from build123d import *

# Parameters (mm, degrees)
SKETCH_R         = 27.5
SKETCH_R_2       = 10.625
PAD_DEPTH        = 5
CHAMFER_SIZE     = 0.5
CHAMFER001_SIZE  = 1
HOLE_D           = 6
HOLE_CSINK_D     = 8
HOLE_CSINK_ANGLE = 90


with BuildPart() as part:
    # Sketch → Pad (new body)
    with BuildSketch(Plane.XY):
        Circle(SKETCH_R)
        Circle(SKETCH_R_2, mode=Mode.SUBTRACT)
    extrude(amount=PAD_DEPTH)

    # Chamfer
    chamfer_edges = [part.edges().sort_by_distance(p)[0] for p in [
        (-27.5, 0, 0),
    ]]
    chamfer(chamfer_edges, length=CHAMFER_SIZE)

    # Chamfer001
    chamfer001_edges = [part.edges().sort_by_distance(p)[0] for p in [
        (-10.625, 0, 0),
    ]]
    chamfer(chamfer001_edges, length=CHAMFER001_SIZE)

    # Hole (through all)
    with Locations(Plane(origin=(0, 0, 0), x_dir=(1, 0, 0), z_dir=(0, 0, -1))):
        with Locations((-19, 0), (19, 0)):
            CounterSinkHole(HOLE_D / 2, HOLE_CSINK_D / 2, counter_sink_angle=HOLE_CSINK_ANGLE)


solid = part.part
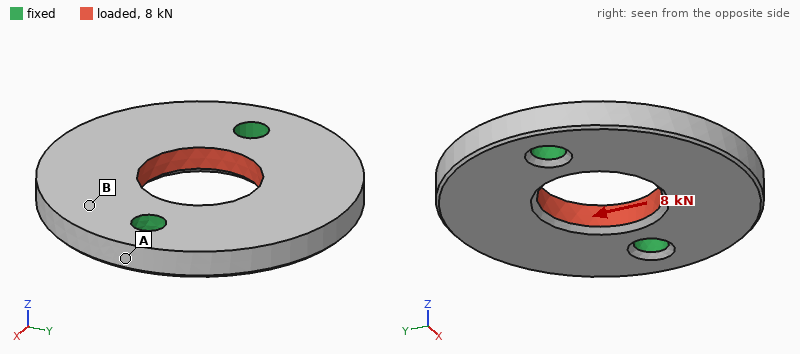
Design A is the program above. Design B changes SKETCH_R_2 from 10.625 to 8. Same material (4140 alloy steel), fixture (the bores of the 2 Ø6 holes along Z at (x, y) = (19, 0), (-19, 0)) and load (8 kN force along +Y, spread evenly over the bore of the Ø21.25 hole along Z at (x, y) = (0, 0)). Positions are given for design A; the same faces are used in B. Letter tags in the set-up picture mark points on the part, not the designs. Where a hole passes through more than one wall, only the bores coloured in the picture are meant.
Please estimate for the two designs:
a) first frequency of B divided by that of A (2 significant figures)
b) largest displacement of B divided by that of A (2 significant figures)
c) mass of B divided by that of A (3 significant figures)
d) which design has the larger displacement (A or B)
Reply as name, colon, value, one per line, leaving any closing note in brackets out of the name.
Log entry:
first frequency of B divided by that of A: 1.0
largest displacement of B divided by that of A: 0.89
mass of B divided by that of A: 1.08
which design has the larger displacement: A
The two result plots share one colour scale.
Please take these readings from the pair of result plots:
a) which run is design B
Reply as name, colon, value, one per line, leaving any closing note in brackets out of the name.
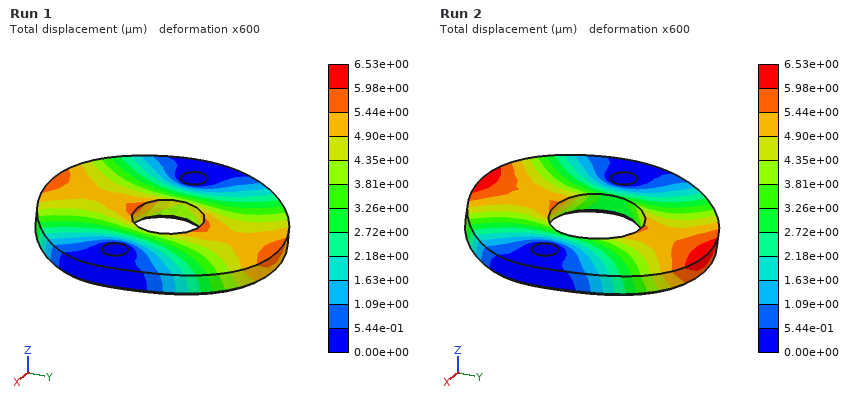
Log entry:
which run is design B: Run 1
